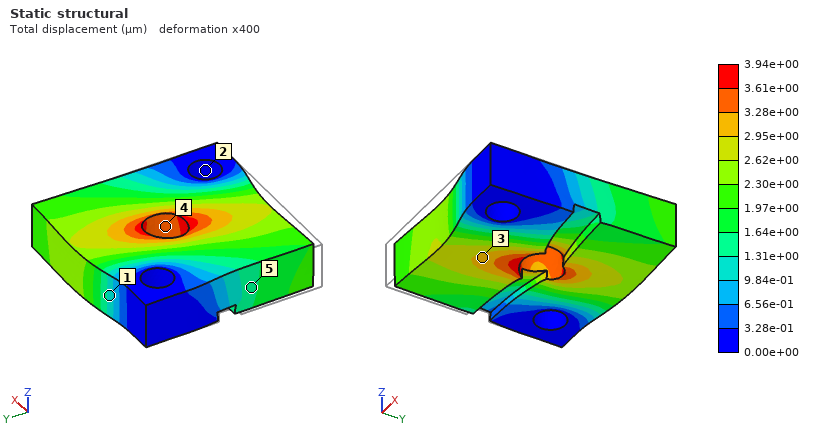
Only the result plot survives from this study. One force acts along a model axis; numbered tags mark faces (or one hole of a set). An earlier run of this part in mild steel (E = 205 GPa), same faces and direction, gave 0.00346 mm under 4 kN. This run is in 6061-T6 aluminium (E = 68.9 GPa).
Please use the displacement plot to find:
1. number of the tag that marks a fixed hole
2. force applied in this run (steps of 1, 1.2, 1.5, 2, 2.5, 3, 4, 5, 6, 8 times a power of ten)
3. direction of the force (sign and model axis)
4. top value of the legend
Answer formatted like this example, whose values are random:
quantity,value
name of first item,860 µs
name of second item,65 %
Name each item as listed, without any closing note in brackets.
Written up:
quantity,value
number of the tag that marks a fixed hole,2
force applied in this run,1.5 kN
direction of the force,+Y
top value of the legend,3.94e+00 µm
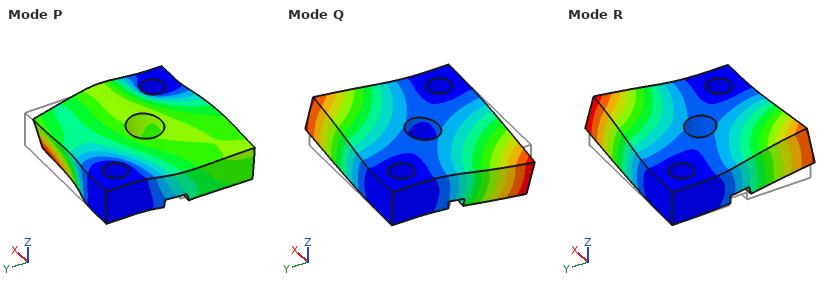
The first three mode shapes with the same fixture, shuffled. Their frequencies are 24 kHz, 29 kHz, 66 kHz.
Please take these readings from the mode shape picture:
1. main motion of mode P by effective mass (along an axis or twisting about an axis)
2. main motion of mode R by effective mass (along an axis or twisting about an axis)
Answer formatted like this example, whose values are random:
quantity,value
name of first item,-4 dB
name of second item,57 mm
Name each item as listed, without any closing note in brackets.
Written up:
quantity,value
main motion of mode P by effective mass,along Y
main motion of mode R by effective mass,along Z
